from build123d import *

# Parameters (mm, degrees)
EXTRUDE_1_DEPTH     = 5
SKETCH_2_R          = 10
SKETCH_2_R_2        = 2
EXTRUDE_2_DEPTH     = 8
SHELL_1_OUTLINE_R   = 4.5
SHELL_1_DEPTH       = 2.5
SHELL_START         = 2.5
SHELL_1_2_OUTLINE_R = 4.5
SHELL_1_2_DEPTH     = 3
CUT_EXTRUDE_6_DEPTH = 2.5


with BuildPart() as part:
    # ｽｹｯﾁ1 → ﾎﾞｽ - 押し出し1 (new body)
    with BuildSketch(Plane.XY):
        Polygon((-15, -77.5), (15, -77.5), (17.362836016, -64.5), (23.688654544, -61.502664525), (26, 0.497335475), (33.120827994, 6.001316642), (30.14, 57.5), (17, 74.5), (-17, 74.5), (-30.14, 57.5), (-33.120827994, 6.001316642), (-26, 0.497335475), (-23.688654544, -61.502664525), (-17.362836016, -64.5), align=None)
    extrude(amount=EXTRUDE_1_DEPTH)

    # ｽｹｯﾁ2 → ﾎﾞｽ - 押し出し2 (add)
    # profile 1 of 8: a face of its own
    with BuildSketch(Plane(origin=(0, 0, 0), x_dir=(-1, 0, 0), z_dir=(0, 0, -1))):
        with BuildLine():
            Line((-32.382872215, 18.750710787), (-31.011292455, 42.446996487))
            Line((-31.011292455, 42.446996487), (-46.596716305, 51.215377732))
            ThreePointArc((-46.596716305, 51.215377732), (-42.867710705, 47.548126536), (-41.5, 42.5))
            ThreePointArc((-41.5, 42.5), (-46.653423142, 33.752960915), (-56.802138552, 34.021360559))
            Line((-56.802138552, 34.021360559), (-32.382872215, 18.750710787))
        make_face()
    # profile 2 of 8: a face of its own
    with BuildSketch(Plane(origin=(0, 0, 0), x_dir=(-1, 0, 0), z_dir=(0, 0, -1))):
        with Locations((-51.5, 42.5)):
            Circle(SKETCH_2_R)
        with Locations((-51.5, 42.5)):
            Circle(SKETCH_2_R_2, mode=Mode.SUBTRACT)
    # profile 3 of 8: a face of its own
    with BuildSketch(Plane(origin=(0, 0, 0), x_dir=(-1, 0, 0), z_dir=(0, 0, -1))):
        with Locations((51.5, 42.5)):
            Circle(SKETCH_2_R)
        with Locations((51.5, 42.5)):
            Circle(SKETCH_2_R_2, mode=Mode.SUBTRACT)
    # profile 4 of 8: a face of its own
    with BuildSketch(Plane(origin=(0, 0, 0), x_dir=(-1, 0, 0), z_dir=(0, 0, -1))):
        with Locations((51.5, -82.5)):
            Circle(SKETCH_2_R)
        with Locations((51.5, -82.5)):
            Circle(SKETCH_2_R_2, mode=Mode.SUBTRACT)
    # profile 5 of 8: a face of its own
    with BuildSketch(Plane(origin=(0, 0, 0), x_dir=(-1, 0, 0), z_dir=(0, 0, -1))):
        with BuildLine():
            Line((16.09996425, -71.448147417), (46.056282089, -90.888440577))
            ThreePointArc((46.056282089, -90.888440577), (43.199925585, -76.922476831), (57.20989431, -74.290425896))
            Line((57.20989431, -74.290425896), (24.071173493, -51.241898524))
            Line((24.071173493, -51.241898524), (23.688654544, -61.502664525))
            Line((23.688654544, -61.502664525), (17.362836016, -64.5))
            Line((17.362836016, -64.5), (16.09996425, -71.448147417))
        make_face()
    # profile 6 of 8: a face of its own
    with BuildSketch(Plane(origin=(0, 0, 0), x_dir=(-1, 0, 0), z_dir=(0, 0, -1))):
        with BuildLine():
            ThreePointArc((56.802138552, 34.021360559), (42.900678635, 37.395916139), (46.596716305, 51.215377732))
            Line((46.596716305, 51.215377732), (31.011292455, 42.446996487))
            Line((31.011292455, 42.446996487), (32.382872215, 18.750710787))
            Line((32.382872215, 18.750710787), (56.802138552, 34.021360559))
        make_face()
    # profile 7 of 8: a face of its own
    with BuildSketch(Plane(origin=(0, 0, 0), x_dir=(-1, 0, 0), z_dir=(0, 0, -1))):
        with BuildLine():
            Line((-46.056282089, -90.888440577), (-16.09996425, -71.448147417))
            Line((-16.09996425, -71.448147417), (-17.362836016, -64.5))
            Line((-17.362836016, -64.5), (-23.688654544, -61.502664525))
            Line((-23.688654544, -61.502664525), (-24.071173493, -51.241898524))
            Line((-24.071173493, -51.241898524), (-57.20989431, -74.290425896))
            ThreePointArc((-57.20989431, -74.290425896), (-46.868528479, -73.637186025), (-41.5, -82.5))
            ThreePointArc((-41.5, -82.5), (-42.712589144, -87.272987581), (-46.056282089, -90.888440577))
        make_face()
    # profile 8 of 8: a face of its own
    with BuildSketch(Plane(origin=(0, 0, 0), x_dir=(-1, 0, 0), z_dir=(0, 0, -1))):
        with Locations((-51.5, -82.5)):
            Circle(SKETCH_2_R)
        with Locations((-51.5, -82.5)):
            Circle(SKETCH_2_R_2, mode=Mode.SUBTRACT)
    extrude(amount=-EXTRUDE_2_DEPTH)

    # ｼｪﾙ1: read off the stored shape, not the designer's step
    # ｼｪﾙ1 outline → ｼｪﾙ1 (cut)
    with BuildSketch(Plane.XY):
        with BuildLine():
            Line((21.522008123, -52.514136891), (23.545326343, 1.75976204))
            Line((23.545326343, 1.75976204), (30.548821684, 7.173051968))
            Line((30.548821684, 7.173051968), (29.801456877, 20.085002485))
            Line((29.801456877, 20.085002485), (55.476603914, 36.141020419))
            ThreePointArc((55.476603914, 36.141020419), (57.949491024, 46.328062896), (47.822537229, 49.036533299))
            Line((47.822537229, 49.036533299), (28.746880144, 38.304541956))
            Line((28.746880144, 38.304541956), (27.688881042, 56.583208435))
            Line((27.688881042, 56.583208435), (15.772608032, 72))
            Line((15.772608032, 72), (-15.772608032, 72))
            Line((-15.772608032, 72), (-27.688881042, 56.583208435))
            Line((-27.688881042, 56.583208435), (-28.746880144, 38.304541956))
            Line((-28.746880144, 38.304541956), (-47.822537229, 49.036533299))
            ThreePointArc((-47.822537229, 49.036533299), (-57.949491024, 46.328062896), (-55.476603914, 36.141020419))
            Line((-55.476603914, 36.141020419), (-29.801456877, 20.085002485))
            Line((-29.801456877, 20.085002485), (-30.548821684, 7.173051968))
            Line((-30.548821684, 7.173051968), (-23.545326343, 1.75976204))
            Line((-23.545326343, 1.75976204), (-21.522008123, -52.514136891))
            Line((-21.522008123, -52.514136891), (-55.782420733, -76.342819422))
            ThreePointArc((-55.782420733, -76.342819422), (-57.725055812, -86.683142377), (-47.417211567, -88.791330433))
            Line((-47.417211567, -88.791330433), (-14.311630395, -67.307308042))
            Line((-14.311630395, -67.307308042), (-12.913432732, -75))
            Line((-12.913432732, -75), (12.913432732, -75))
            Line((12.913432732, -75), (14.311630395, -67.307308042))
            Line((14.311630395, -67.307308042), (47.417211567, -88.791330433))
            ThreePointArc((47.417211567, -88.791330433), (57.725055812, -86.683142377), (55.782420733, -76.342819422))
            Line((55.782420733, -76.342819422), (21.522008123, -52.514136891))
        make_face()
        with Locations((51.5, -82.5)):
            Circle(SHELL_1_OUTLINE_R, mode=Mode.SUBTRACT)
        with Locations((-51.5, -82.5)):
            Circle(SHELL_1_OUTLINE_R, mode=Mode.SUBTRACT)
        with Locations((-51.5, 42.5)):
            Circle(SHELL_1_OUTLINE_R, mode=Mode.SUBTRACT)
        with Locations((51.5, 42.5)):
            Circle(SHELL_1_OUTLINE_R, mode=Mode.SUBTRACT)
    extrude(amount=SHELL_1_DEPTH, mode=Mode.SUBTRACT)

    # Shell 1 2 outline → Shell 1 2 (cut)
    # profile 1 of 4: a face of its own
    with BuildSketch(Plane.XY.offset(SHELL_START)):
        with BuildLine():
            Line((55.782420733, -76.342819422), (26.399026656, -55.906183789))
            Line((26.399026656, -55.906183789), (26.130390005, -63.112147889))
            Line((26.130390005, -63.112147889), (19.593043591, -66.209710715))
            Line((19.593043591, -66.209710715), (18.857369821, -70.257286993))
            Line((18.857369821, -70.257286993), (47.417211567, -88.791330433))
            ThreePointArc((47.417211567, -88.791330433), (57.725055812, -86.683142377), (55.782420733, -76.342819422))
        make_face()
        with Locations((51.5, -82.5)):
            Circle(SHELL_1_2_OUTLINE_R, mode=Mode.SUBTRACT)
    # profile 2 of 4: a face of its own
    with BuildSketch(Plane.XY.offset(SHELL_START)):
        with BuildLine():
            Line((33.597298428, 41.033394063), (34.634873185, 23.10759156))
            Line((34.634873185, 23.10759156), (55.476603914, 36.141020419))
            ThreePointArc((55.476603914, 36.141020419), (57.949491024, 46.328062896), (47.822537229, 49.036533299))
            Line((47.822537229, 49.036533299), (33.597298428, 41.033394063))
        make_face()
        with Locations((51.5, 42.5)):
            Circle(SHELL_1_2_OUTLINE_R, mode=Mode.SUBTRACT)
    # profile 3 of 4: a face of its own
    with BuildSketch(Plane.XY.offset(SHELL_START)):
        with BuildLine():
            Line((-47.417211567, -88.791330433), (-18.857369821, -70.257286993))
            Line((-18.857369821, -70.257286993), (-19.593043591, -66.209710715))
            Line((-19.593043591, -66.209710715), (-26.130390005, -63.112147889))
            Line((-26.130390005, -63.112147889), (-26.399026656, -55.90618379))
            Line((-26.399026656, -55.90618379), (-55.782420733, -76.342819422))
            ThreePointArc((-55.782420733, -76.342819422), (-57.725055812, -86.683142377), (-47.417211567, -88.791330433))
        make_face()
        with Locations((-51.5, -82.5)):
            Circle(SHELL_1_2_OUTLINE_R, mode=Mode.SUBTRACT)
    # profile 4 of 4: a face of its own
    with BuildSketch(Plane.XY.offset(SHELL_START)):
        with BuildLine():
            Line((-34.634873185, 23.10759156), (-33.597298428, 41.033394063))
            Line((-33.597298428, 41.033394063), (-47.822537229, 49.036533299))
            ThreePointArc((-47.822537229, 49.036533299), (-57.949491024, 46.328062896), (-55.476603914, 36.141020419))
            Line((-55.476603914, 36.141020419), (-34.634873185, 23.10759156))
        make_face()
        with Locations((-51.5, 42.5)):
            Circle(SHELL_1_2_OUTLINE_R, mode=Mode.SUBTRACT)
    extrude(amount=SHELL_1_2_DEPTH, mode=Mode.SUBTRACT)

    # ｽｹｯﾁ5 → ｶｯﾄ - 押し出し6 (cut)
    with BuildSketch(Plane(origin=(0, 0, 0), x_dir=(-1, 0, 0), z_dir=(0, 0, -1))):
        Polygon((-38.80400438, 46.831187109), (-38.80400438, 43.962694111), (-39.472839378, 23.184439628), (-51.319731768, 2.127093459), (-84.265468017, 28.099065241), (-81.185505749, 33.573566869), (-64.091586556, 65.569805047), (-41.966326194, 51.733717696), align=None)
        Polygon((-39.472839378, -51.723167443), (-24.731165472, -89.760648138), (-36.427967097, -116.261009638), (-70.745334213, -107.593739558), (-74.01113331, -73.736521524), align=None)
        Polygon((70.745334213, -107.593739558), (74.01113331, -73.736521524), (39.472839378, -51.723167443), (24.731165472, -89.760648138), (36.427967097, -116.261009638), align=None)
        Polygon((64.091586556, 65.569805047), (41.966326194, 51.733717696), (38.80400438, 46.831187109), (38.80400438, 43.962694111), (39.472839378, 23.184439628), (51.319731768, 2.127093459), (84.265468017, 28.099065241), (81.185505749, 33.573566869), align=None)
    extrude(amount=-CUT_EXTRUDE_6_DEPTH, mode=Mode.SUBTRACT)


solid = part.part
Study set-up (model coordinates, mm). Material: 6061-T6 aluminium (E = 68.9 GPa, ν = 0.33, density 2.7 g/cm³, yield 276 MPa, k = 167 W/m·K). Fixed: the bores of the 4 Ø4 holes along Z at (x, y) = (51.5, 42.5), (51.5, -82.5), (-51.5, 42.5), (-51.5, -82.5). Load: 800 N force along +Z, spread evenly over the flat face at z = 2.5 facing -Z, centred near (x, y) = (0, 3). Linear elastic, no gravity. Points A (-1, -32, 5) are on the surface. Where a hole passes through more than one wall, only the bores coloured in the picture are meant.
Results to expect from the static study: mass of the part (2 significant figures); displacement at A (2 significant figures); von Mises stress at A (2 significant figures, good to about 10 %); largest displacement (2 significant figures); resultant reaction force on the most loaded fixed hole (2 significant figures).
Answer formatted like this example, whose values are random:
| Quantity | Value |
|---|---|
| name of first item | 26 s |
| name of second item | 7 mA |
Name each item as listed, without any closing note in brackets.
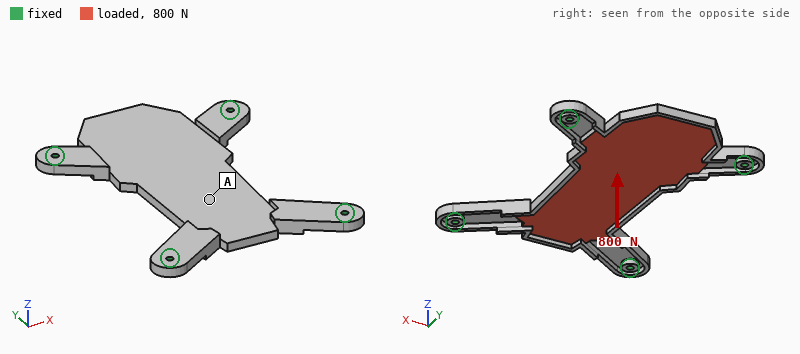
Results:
| Quantity | Value |
|---|---|
| mass of the part | 92 g |
| displacement at A | 0.34 mm |
| von Mises stress at A | 22 MPa |
| largest displacement | 0.37 mm |
| resultant reaction force on the most loaded fixed hole | 1.2 kN |
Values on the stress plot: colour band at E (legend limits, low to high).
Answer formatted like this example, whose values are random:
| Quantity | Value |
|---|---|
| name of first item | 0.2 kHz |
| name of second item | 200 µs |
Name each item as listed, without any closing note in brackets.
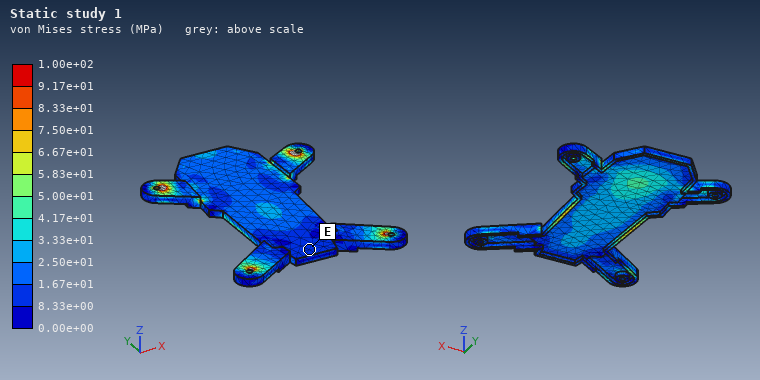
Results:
| Quantity | Value |
|---|---|
| colour band at E | 8.33e+00 to 1.67e+01 MPa |
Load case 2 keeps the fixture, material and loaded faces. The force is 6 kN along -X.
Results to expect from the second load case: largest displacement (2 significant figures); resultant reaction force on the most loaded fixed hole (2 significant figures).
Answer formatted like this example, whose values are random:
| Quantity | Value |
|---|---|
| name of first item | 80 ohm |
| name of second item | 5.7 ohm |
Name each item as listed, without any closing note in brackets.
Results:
| Quantity | Value |
|---|---|
| largest displacement | 77 µm |
| resultant reaction force on the most loaded fixed hole | 2.2 kN |
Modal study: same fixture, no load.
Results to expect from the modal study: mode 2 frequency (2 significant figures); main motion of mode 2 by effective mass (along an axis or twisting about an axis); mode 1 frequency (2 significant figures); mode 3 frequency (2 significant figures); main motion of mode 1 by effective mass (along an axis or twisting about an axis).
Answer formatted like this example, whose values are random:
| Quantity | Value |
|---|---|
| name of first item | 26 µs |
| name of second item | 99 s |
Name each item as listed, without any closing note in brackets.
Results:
| Quantity | Value |
|---|---|
| mode 2 frequency | 1200 Hz |
| main motion of mode 2 by effective mass | along Z |
| mode 1 frequency | 1100 Hz |
| mode 3 frequency | 1800 Hz |
| main motion of mode 1 by effective mass | along Z |
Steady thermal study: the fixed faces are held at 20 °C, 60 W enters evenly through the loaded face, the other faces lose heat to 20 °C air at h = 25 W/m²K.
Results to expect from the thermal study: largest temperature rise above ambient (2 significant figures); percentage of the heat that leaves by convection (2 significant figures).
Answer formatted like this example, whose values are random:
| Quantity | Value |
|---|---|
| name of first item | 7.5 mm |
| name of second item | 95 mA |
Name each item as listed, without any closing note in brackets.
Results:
| Quantity | Value |
|---|---|
| largest temperature rise above ambient | 47 K |
| percentage of the heat that leaves by convection | 25 % |
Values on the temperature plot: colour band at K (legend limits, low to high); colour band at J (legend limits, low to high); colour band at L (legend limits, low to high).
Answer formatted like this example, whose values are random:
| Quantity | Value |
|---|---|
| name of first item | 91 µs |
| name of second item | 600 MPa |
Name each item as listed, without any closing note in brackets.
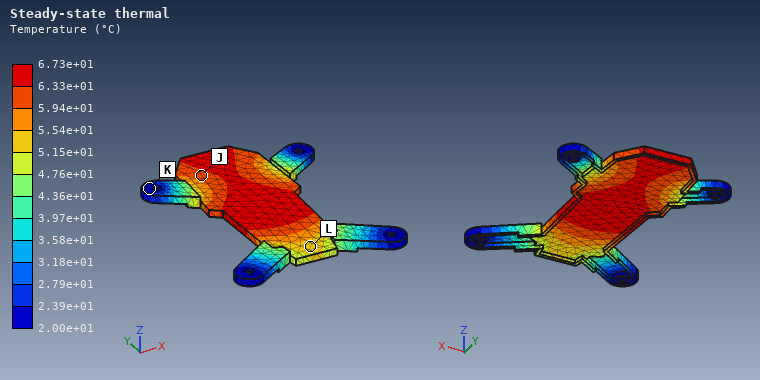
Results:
| Quantity | Value |
|---|---|
| colour band at K | 2.00e+01 to 2.39e+01 °C |
| colour band at J | 5.94e+01 to 6.33e+01 °C |
| colour band at L | 5.15e+01 to 5.54e+01 °C |
